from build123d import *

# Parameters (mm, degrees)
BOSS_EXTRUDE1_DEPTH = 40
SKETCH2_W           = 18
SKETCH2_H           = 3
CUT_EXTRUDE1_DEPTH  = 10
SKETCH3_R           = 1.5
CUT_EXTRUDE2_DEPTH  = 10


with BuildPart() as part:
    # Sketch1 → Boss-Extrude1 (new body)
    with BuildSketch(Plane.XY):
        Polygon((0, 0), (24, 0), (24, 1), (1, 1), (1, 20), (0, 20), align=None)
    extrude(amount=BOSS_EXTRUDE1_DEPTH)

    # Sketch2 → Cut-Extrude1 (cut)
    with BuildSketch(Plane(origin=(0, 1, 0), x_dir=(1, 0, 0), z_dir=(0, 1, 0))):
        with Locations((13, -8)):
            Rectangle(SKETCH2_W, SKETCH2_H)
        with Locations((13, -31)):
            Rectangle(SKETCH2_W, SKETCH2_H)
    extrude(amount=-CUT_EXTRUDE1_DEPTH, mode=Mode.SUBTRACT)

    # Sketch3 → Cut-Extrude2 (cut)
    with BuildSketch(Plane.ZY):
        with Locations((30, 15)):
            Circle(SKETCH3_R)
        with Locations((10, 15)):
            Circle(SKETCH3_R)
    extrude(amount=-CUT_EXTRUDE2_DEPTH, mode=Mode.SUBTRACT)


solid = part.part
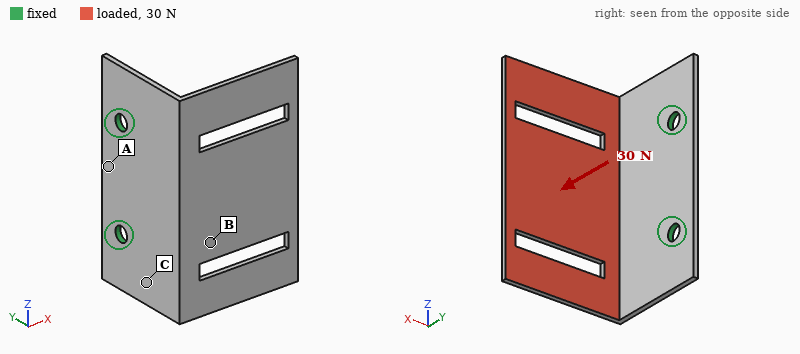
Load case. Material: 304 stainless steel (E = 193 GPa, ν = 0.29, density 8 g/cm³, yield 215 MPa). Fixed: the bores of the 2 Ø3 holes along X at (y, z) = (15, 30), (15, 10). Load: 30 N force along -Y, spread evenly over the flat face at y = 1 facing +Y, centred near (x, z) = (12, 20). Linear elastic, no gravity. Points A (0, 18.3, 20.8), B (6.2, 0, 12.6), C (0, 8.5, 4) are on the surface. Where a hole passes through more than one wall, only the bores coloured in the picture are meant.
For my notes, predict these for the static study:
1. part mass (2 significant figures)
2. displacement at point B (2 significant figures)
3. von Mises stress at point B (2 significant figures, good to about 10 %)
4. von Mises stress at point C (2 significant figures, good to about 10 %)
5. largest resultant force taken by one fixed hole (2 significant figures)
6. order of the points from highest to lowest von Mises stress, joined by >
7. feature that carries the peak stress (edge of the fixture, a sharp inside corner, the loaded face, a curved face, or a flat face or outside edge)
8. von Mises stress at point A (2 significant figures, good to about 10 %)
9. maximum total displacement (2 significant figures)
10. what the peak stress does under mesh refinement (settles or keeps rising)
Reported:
13 g
0.080 mm
35 MPa
49 MPa
15 N
C > B > A
edge of the fixture
11 MPa
0.27 mm
keeps rising
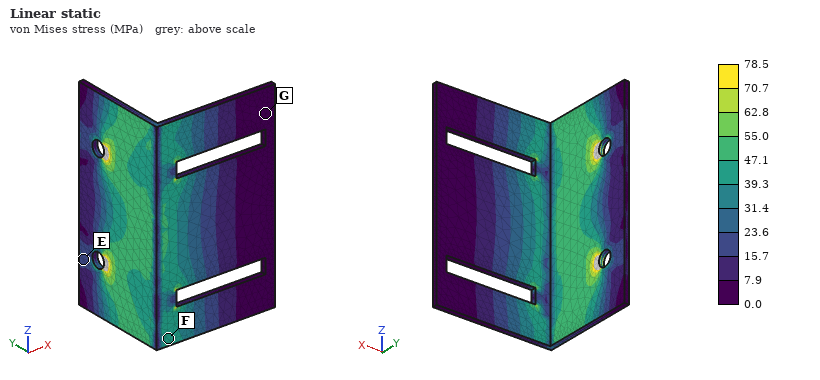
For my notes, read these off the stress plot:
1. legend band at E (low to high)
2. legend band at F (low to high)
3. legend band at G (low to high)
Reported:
15.7 to 23.6 MPa
39.3 to 47.1 MPa
0.0 to 7.9 MPa
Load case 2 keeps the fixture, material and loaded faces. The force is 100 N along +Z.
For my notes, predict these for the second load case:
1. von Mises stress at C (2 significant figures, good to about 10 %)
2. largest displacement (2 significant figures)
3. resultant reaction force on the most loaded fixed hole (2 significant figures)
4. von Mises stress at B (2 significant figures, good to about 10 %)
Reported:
53 MPa
0.21 mm
92 N
36 MPa
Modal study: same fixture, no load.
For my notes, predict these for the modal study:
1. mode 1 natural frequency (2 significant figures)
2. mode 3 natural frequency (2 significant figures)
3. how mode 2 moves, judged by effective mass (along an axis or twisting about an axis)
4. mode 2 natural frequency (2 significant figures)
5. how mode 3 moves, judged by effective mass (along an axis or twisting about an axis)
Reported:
750 Hz
2200 Hz
along Z
1400 Hz
along X
